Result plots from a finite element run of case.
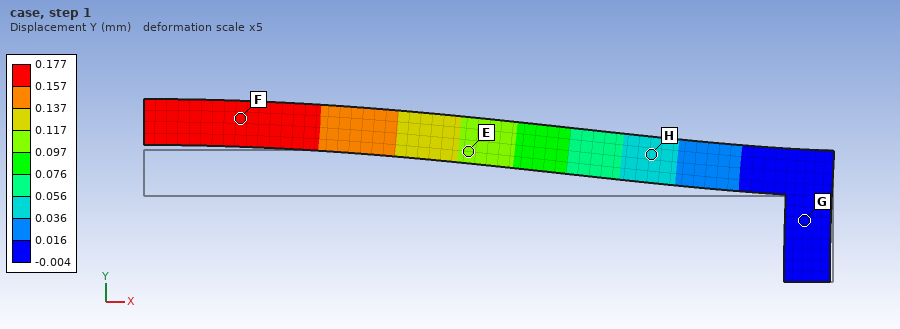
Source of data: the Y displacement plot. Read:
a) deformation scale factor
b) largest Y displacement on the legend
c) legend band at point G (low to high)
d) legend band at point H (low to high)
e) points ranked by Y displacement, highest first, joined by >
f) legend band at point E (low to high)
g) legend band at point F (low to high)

5
0.177 mm
-0.004 to 0.016 mm
0.036 to 0.056 mm
F > E > H > G
0.097 to 0.117 mm
0.157 to 0.177 mm
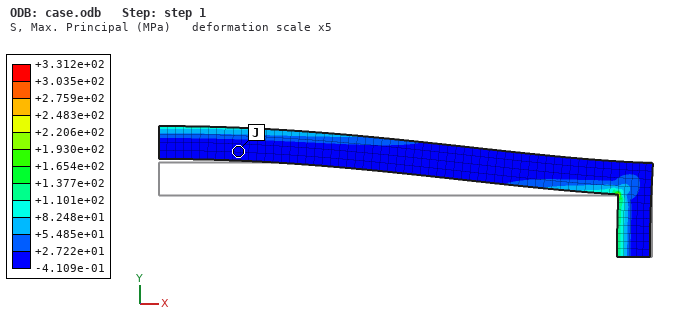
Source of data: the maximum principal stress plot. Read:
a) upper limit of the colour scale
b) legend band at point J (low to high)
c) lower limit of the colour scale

+3.312e+02 MPa
-4.109e-01 to +2.722e+01 MPa
-4.109e-01 MPa
